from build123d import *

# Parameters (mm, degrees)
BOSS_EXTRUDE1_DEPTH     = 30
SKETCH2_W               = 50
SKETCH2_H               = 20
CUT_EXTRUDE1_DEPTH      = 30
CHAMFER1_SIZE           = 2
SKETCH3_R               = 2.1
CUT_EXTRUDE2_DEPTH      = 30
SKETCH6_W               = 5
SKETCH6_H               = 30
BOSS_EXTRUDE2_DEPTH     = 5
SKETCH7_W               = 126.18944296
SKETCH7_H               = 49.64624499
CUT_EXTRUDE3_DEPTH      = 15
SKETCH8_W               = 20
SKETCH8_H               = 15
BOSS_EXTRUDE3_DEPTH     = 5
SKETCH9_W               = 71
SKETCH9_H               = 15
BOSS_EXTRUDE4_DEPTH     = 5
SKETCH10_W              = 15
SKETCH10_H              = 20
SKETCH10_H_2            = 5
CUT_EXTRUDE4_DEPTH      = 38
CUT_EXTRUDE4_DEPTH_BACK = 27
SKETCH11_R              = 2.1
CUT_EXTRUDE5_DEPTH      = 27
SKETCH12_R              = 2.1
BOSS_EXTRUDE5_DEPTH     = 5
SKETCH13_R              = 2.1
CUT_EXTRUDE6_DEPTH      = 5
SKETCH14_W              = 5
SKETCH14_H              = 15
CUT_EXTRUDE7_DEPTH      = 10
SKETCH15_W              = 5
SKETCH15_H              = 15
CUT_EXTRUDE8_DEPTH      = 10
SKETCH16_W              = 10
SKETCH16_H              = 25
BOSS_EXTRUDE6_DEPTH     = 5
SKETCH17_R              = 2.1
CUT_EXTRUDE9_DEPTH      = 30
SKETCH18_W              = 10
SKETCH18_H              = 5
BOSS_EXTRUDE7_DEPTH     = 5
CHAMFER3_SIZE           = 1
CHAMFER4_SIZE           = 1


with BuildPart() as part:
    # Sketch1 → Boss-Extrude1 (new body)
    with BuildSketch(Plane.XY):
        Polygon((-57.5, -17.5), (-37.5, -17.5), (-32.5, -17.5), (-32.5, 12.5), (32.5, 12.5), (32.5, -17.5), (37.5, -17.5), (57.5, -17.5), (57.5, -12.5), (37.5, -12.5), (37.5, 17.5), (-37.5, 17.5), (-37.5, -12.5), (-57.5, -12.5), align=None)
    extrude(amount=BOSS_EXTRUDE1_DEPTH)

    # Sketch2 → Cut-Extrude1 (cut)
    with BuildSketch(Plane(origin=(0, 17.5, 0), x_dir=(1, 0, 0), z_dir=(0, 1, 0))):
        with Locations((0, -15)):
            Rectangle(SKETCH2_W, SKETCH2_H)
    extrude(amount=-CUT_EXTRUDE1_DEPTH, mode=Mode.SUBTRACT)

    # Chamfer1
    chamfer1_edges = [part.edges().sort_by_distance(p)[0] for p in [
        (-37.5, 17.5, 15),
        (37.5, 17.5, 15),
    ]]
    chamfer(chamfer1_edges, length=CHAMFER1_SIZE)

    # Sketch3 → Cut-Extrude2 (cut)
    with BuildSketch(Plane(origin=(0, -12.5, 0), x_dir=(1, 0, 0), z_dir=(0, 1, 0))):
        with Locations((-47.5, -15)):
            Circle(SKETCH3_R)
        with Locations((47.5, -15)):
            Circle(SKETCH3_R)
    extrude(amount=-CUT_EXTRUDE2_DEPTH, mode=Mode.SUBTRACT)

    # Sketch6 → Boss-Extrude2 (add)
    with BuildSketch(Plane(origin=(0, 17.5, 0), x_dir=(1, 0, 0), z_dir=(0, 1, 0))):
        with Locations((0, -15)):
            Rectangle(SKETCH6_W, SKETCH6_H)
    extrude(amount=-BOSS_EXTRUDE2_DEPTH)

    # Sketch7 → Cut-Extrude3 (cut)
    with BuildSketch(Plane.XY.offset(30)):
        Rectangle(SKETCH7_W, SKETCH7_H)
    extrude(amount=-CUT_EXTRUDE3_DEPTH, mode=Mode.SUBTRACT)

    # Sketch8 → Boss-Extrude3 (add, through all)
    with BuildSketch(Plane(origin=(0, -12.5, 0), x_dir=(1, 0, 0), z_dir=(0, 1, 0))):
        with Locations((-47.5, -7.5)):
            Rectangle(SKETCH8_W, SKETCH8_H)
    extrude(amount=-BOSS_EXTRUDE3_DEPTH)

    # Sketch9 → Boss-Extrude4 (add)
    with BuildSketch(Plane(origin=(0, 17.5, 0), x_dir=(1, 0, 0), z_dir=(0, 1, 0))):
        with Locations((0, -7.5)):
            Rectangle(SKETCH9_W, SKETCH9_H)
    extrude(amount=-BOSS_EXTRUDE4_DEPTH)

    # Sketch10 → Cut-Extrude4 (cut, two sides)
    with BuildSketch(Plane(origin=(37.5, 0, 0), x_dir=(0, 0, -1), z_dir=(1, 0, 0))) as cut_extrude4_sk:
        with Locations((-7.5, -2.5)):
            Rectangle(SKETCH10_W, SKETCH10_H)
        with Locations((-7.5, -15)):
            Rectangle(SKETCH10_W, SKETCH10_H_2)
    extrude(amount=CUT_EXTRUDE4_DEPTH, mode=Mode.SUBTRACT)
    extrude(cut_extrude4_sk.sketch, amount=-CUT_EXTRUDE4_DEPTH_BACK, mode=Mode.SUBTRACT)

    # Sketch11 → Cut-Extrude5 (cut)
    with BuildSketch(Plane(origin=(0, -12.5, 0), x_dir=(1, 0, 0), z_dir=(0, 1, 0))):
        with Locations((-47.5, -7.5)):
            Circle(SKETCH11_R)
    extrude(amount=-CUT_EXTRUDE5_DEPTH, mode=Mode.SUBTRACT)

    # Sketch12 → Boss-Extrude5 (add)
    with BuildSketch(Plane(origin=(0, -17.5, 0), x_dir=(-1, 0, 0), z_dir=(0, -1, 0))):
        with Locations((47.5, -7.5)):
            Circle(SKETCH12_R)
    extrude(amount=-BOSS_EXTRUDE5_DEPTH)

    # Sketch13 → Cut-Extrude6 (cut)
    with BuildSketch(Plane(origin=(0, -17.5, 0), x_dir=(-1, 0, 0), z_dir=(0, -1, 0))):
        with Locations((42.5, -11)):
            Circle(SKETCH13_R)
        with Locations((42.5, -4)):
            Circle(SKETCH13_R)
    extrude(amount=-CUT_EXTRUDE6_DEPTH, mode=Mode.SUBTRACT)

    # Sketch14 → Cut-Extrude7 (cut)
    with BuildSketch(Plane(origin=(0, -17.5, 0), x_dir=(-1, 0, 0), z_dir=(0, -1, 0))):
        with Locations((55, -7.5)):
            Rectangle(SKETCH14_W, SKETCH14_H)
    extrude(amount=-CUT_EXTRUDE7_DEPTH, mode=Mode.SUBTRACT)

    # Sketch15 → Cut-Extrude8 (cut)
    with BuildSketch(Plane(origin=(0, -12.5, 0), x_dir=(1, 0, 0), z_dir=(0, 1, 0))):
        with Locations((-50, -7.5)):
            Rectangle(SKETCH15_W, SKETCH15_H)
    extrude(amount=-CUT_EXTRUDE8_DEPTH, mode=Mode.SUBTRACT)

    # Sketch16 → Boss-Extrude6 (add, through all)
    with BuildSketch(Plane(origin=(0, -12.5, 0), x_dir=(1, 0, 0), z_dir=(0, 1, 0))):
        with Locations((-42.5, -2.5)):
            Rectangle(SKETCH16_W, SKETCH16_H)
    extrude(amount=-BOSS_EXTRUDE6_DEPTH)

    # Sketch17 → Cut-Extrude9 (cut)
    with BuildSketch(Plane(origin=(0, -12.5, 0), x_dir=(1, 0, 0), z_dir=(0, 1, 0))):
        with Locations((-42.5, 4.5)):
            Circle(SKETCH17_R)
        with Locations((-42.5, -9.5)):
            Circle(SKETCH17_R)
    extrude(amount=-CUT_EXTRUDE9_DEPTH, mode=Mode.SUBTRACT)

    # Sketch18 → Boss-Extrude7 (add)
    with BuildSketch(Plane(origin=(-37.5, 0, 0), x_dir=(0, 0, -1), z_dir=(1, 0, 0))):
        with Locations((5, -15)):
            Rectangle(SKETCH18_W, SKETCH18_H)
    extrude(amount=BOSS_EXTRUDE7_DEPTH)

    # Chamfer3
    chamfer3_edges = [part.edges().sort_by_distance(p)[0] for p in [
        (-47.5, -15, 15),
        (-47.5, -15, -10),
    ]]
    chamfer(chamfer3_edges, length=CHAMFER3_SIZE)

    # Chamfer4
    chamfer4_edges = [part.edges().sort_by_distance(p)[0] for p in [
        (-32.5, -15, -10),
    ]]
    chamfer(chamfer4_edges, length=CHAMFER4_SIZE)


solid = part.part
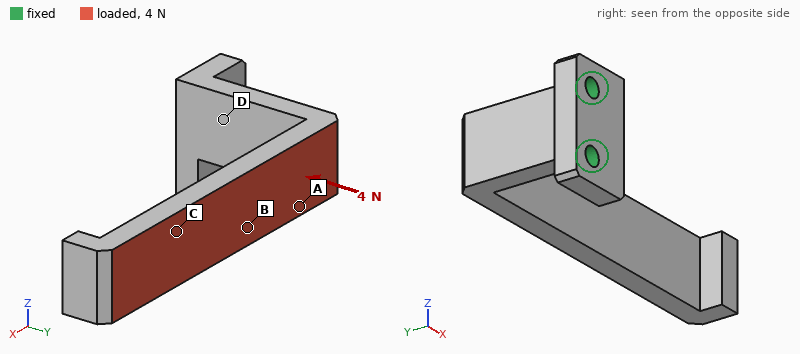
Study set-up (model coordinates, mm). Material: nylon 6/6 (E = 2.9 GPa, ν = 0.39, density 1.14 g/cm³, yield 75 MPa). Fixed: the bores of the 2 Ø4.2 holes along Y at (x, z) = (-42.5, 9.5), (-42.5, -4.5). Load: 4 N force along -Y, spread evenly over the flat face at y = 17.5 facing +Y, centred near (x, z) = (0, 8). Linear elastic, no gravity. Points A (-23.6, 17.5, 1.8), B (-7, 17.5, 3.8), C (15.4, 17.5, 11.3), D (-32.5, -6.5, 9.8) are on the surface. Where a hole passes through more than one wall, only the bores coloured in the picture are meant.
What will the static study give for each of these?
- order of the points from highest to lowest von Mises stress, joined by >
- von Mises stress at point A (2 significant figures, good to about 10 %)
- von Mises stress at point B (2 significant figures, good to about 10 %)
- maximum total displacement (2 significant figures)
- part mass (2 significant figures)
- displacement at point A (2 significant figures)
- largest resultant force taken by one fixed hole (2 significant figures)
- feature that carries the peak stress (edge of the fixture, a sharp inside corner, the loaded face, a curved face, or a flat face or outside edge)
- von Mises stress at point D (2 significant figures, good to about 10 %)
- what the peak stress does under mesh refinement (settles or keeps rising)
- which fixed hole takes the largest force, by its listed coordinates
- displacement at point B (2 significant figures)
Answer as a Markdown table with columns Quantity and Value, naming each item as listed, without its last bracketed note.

| Quantity | Value |
|---|---|
| order of the points from highest to lowest von Mises stress, joined by > | D > A > B > C |
| von Mises stress at point A | 1.6 MPa |
| von Mises stress at point B | 0.82 MPa |
| maximum total displacement | 1.1 mm |
| part mass | 11 g |
| displacement at point A | 0.24 mm |
| largest resultant force taken by one fixed hole | 3.0 N |
| feature that carries the peak stress | edge of the fixture |
| von Mises stress at point D | 2.2 MPa |
| what the peak stress does under mesh refinement | keeps rising |
| which fixed hole takes the largest force, by its listed coordinates | (-42.5, 9.5) |
| displacement at point B | 0.42 mm |
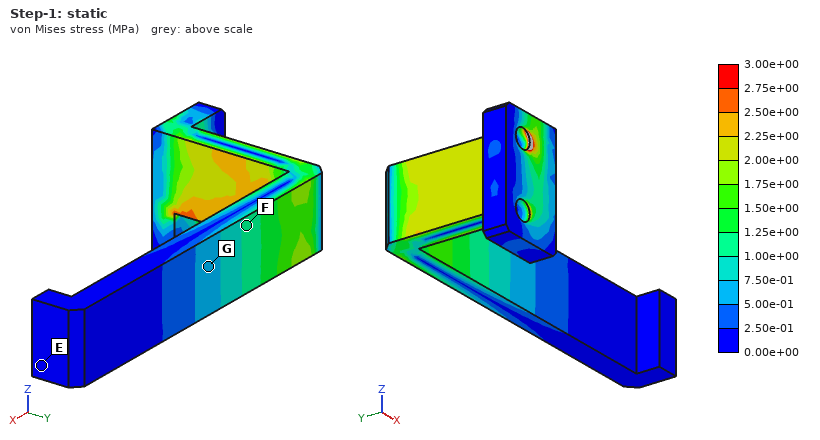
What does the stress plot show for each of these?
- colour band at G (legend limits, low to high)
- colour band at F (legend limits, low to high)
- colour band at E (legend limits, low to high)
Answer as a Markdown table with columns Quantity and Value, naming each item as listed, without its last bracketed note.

| Quantity | Value |
|---|---|
| colour band at G | 5.00e-01 to 7.50e-01 MPa |
| colour band at F | 1.00e+00 to 1.25e+00 MPa |
| colour band at E | 0.00e+00 to 2.50e-01 MPa |
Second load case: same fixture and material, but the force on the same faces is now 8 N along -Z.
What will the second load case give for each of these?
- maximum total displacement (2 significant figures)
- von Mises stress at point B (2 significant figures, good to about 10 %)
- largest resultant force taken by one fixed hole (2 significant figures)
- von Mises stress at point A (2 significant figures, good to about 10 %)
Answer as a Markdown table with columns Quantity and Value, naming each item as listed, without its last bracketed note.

| Quantity | Value |
|---|---|
| maximum total displacement | 1.1 mm |
| von Mises stress at point B | 0.43 MPa |
| largest resultant force taken by one fixed hole | 29 N |
| von Mises stress at point A | 0.66 MPa |
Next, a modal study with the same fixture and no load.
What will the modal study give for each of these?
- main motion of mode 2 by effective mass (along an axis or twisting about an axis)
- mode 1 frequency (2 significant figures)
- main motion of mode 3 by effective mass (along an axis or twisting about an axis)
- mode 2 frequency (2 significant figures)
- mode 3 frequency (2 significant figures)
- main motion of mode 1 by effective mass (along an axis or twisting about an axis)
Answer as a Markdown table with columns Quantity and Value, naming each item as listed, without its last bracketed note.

| Quantity | Value |
|---|---|
| main motion of mode 2 by effective mass | along Z |
| mode 1 frequency | 130 Hz |
| main motion of mode 3 by effective mass | along X |
| mode 2 frequency | 190 Hz |
| mode 3 frequency | 510 Hz |
| main motion of mode 1 by effective mass | along Y |
